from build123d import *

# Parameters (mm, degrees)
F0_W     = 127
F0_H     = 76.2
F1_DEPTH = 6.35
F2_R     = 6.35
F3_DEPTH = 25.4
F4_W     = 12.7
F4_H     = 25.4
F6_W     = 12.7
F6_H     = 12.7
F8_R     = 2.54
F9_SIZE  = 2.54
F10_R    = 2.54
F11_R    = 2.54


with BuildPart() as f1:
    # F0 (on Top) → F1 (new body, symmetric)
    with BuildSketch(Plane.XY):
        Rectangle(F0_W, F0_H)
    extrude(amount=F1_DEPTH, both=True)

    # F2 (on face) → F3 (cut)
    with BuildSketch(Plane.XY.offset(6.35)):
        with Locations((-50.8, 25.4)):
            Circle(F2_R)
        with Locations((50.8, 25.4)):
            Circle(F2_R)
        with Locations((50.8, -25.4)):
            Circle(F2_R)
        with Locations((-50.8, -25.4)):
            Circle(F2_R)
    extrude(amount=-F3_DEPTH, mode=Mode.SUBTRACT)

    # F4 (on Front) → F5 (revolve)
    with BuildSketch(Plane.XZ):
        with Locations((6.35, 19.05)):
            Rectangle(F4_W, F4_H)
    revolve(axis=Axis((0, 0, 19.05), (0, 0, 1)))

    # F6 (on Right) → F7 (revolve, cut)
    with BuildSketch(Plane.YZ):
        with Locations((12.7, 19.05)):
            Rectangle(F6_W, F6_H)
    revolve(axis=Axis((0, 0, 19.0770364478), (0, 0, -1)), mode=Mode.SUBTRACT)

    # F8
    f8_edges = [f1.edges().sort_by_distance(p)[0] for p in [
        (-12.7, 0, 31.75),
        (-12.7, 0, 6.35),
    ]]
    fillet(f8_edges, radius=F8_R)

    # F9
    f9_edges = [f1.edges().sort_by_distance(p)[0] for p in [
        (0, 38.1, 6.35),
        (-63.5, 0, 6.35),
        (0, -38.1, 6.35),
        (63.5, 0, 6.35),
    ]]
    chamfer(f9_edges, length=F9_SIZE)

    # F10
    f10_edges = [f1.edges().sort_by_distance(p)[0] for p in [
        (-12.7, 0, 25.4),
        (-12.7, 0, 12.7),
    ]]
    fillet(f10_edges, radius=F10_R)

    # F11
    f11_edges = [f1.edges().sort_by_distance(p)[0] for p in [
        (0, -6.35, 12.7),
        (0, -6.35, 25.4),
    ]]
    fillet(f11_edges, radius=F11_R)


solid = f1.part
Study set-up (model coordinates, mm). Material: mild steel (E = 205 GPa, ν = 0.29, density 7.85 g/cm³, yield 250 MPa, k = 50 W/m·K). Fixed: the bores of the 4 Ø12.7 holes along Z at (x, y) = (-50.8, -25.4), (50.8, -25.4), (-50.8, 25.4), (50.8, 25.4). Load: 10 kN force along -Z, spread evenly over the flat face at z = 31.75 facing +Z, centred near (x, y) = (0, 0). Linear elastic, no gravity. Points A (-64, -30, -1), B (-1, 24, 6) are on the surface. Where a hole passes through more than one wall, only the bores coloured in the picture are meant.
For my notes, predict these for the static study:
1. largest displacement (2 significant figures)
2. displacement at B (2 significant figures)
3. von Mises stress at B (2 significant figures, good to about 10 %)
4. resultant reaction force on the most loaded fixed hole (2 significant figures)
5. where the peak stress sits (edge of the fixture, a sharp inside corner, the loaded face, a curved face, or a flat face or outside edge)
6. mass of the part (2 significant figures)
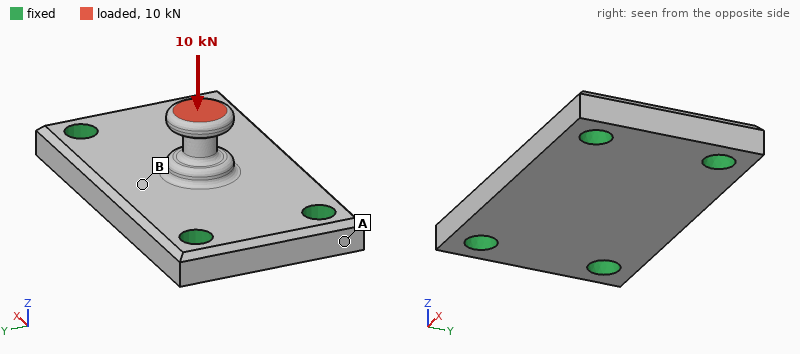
28 µm
17 µm
32 MPa
2.5 kN
a curved face
970 g
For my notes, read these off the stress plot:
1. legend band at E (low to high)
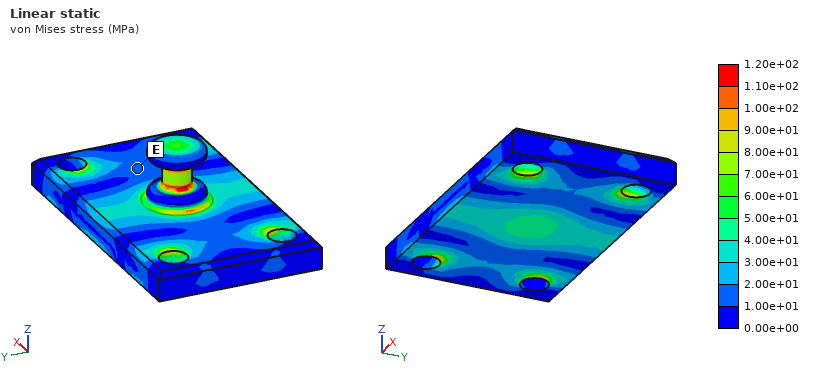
1.00e+01 to 2.00e+01 MPa
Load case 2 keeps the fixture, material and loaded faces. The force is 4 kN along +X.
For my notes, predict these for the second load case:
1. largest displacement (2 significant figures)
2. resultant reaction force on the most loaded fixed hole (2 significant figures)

72 µm
1.4 kN
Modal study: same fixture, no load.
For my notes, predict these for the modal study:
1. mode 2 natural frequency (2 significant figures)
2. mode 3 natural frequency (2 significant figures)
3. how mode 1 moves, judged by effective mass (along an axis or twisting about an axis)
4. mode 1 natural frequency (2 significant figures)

7100 Hz
8700 Hz
along Z
6000 Hz
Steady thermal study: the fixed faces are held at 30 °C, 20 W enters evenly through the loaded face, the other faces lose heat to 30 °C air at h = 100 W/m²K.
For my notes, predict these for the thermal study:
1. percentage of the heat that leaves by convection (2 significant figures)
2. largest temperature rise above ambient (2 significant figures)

52 %
52 K
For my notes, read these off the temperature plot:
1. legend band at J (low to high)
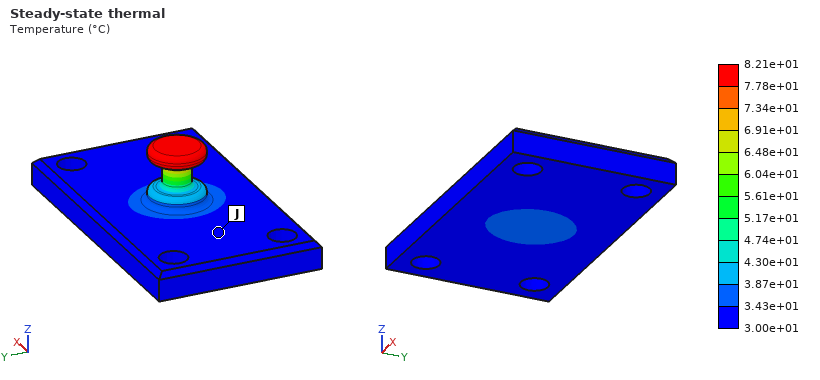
3.00e+01 to 3.43e+01 °C
